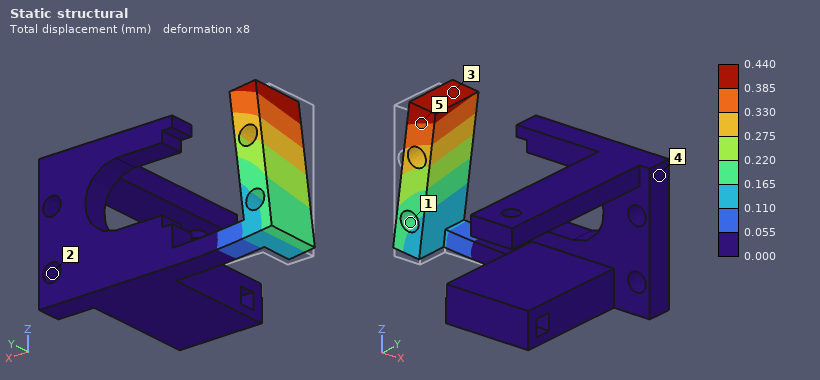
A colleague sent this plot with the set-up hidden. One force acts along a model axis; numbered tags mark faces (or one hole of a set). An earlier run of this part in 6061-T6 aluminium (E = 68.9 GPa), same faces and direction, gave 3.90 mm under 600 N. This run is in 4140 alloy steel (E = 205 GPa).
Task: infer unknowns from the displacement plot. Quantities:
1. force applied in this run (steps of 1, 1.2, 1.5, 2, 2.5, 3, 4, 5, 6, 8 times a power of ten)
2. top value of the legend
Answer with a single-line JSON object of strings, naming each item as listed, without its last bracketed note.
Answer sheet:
{"force applied in this run": "200 N", "top value of the legend": "0.440 mm"}
